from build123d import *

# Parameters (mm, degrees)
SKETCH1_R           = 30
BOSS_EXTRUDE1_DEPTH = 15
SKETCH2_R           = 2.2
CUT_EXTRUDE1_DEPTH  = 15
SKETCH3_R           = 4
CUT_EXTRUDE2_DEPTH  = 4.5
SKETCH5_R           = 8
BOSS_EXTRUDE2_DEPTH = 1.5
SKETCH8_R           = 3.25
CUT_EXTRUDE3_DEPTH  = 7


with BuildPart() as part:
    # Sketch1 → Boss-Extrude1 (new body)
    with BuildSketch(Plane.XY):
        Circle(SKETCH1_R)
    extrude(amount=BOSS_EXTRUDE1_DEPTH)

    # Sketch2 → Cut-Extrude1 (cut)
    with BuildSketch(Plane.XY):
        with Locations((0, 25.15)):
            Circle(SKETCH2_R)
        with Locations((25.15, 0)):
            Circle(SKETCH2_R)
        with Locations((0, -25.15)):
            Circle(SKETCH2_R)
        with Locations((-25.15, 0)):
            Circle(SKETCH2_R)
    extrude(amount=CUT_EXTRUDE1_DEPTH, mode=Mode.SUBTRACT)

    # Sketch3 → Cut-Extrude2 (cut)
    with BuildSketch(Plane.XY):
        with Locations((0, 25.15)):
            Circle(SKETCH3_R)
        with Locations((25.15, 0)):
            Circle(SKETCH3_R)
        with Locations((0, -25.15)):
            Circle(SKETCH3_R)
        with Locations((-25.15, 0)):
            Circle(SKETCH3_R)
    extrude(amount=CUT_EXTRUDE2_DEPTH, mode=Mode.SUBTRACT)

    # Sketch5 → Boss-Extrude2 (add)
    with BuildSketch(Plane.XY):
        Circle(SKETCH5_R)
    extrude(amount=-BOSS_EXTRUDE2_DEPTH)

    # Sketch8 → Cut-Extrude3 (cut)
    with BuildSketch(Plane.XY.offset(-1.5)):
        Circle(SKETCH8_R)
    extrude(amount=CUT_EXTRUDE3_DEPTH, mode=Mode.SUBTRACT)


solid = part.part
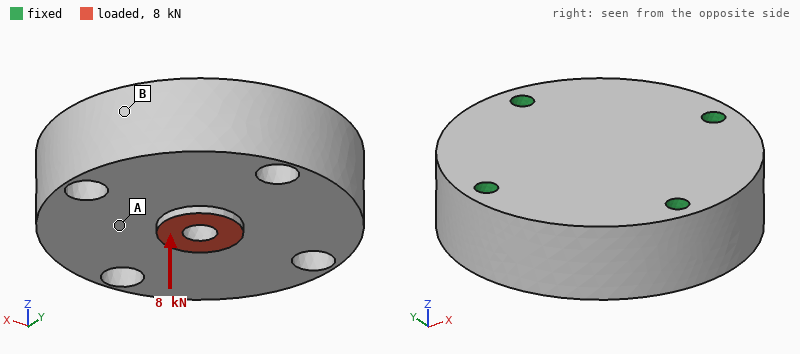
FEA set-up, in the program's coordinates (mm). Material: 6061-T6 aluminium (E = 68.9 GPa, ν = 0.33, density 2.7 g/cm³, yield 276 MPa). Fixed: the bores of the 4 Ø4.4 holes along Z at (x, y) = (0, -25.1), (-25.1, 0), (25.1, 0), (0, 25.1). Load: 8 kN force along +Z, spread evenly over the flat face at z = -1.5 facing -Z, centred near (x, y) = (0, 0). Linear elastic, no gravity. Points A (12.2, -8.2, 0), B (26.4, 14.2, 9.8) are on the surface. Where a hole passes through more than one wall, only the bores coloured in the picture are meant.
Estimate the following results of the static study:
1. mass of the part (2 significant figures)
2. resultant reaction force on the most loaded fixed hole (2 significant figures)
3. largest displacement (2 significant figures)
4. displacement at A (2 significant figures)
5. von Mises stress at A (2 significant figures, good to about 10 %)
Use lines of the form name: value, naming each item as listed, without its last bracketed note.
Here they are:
mass of the part: 110 g
resultant reaction force on the most loaded fixed hole: 2.2 kN
largest displacement: 16 µm
displacement at A: 6.8 µm
von Mises stress at A: 14 MPa
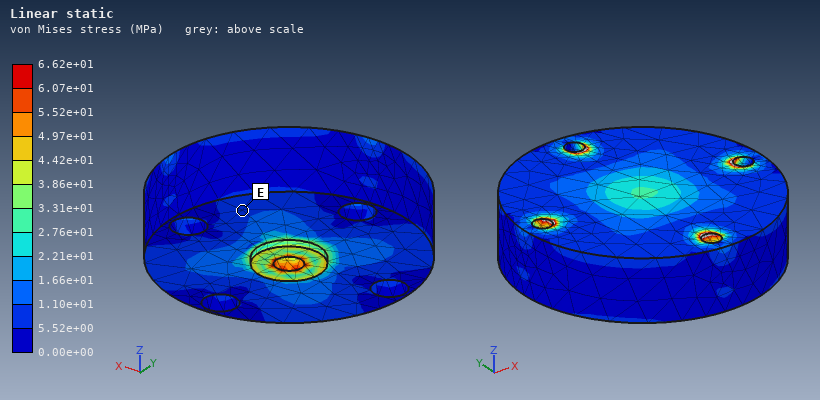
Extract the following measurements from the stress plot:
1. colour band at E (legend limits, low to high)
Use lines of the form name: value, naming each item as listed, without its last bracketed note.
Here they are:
colour band at E: 5.52e+00 to 1.10e+01 MPa
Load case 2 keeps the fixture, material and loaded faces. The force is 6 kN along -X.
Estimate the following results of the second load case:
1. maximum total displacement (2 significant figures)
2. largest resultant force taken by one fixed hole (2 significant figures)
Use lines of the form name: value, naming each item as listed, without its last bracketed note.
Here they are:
maximum total displacement: 13 µm
largest resultant force taken by one fixed hole: 2.4 kN
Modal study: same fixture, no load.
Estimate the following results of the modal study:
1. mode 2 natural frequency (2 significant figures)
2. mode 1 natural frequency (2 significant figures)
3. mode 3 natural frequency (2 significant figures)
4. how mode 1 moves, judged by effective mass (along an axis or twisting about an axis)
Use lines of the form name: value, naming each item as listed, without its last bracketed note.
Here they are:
mode 2 natural frequency: 25 kHz
mode 1 natural frequency: 23 kHz
mode 3 natural frequency: 26 kHz
how mode 1 moves, judged by effective mass: along Z
